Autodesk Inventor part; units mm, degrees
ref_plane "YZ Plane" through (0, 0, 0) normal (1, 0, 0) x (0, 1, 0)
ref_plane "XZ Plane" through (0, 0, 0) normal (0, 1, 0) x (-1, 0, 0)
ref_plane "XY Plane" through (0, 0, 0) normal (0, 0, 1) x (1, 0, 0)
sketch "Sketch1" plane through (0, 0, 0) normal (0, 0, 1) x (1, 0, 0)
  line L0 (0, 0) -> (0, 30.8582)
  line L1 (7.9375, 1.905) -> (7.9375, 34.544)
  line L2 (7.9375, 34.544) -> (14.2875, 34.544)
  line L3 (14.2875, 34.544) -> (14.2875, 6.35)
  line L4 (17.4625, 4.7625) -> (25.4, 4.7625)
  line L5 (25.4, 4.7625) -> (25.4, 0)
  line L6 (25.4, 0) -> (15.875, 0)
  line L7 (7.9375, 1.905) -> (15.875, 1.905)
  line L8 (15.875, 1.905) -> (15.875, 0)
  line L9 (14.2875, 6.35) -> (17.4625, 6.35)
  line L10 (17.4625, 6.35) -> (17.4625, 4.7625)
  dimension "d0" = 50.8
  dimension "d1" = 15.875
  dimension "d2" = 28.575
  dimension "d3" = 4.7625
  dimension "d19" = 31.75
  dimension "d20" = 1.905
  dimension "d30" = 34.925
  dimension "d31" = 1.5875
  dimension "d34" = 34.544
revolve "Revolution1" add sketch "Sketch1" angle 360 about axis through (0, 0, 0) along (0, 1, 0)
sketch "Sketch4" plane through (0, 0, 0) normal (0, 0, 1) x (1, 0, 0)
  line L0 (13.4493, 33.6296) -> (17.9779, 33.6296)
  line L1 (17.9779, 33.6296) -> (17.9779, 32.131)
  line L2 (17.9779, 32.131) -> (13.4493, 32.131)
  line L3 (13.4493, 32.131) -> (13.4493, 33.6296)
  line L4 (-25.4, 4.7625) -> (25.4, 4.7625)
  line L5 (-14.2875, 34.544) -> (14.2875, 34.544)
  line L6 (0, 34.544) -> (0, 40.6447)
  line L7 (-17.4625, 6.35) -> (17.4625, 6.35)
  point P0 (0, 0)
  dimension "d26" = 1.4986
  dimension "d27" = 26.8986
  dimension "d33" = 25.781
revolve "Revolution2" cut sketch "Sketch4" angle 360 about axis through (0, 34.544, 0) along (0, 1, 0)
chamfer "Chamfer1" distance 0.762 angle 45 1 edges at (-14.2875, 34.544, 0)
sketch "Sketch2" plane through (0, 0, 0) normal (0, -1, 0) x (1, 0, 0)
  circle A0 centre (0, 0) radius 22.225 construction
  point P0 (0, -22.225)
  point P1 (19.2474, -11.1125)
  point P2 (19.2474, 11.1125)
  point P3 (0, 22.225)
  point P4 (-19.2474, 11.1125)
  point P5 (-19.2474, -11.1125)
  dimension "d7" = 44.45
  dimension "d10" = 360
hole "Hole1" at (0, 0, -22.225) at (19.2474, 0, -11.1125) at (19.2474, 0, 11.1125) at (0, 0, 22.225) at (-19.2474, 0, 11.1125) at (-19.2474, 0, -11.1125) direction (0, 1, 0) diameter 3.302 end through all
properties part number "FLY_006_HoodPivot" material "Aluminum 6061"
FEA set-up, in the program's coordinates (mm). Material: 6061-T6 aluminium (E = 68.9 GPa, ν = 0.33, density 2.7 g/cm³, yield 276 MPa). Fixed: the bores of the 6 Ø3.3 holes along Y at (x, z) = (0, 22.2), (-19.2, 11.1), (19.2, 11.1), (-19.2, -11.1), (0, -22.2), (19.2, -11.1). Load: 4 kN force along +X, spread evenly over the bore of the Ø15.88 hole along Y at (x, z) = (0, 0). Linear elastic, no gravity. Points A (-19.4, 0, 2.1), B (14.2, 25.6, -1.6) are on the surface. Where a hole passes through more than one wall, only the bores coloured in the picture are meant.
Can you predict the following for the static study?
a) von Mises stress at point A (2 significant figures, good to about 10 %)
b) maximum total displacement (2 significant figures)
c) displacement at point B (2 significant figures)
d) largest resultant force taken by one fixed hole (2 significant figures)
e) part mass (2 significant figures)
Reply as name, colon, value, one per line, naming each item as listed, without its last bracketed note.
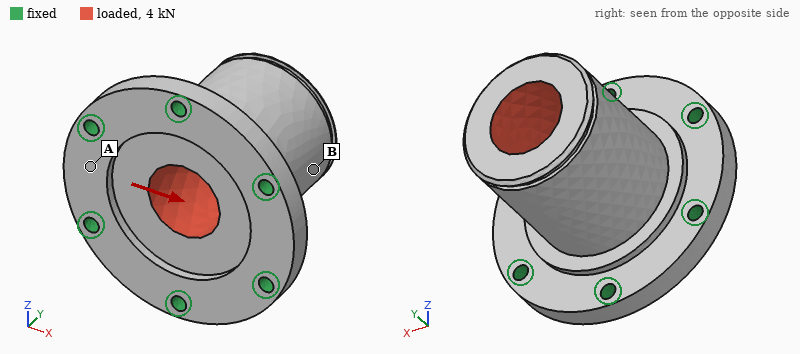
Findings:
von Mises stress at point A: 21 MPa
maximum total displacement: 39 µm
displacement at point B: 30 µm
largest resultant force taken by one fixed hole: 1.3 kN
part mass: 56 g
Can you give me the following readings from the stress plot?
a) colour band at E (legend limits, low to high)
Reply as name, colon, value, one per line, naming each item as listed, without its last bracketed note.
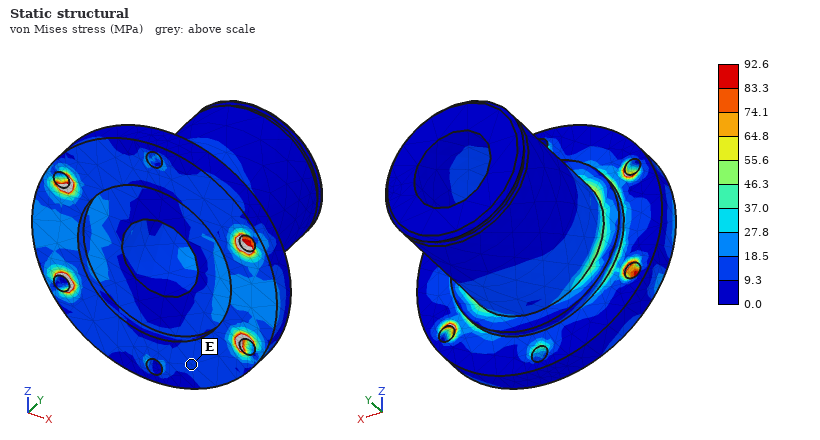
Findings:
colour band at E: 9.3 to 18.5 MPa
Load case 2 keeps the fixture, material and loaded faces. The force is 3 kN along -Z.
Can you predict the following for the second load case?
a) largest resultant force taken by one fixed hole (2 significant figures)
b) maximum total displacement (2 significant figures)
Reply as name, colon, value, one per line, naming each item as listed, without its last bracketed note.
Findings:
largest resultant force taken by one fixed hole: 1.2 kN
maximum total displacement: 29 µm
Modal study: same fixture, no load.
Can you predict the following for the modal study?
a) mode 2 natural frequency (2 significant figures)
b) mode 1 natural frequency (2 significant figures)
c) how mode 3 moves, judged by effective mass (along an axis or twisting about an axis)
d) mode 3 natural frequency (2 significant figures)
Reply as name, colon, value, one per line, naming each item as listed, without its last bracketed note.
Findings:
mode 2 natural frequency: 9500 Hz
mode 1 natural frequency: 9500 Hz
how mode 3 moves, judged by effective mass: along Y
mode 3 natural frequency: 15 kHz
